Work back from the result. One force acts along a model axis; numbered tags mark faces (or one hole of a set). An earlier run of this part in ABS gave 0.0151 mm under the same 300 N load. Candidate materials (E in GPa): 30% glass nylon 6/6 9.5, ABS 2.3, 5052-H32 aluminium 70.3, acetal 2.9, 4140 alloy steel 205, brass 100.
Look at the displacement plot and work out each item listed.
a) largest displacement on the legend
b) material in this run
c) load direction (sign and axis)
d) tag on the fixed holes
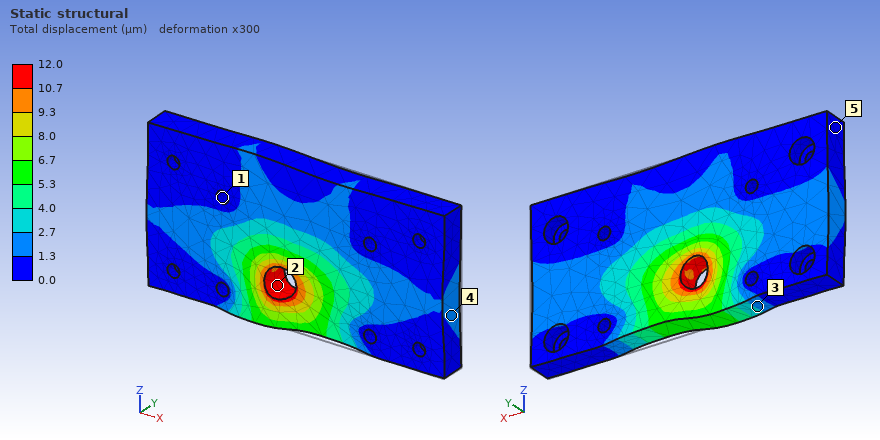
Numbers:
12.0 µm
acetal
-X
1
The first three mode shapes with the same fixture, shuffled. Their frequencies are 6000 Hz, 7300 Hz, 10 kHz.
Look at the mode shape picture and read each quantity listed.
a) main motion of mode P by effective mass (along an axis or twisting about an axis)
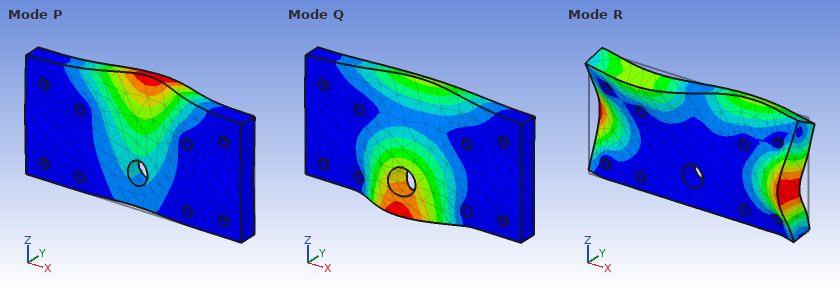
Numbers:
along Y
